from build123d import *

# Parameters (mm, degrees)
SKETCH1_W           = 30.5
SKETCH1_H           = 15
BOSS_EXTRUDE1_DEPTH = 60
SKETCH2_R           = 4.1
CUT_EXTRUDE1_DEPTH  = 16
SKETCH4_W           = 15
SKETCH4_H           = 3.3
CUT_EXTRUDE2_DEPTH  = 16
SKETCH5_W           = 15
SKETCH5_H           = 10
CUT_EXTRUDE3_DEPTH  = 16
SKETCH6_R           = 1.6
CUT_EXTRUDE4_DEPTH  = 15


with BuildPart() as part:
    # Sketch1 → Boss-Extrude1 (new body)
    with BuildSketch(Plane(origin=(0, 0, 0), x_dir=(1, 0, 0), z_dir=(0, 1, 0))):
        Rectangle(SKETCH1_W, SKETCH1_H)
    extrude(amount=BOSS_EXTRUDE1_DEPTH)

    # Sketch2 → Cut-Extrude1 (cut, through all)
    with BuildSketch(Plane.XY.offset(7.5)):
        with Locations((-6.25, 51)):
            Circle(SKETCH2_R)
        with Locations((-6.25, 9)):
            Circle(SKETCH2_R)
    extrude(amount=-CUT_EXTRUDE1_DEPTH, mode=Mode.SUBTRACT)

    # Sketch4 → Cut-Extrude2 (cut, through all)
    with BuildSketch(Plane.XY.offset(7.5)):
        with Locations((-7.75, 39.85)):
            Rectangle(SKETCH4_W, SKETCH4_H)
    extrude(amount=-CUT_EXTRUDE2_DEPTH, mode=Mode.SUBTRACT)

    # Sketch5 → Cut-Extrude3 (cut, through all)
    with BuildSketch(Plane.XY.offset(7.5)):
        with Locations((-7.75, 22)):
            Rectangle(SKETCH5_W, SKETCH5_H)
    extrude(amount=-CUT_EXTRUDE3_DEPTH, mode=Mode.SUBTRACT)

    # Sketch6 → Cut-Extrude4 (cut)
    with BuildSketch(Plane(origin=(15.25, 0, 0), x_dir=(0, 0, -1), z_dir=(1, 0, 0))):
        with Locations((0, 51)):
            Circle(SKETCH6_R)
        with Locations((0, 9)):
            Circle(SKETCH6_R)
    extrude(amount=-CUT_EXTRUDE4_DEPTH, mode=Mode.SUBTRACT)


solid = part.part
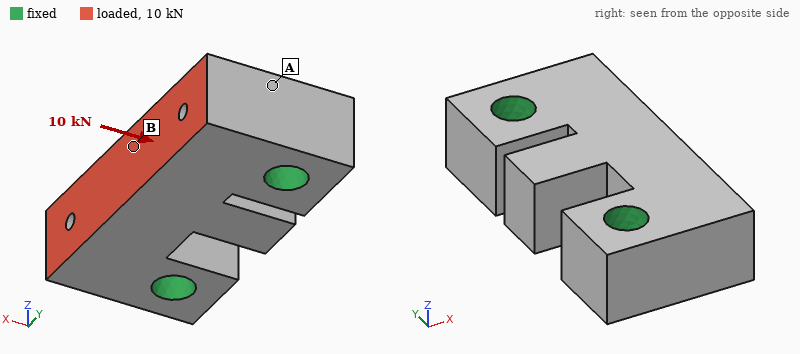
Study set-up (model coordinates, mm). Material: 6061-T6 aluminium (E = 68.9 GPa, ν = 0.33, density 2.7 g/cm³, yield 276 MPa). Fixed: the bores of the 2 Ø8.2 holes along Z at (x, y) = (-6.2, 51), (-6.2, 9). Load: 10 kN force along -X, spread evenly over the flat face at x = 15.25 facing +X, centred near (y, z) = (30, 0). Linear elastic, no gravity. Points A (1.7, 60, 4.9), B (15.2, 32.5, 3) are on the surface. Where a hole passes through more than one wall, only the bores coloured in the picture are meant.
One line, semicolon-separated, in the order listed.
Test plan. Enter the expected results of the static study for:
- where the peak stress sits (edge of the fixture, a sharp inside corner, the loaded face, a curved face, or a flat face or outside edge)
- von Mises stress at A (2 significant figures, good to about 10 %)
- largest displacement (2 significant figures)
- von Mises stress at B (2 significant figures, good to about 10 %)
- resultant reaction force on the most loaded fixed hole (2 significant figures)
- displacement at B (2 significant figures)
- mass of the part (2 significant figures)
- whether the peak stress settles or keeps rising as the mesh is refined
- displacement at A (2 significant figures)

edge of the fixture; 4.6 MPa; 9.4 µm; 17 MPa; 5.3 kN; 8.9 µm; 61 g; keeps rising; 1.4 µm
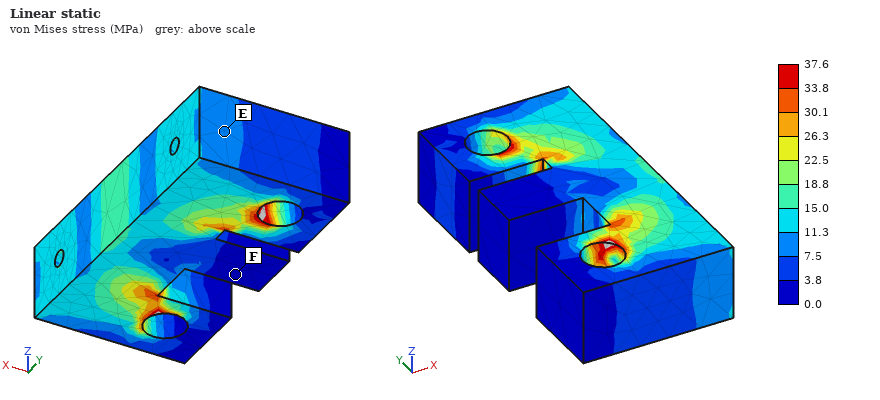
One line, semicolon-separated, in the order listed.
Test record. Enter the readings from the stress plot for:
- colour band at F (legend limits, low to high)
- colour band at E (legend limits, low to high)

0.0 to 3.8 MPa; 7.5 to 11.3 MPa
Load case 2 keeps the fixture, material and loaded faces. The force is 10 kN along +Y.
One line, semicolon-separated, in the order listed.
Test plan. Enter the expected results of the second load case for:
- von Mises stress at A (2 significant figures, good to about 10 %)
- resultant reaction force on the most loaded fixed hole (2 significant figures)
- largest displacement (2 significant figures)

25 MPa; 6.1 kN; 25 µm
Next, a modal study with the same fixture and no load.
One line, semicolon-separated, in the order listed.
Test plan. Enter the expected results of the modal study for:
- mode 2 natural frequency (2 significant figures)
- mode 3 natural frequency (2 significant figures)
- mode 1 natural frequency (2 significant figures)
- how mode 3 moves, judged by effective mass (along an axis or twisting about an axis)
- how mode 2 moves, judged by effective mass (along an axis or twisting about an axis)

17 kHz; 18 kHz; 14 kHz; along Y; along Z
